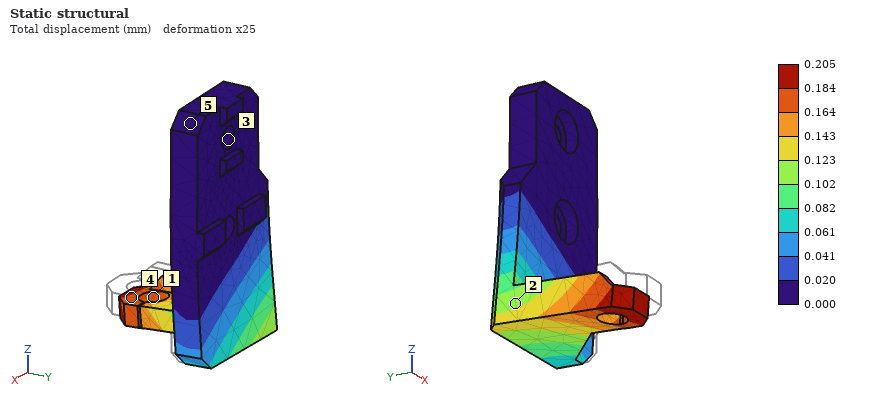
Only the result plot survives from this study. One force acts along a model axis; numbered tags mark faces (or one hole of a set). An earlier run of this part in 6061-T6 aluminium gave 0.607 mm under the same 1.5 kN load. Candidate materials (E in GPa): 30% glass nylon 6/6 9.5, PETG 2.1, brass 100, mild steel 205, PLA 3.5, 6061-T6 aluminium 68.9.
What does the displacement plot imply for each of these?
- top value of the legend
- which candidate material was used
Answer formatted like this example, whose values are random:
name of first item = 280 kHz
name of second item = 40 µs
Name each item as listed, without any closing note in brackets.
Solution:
top value of the legend = 0.205 mm
which candidate material was used = mild steel
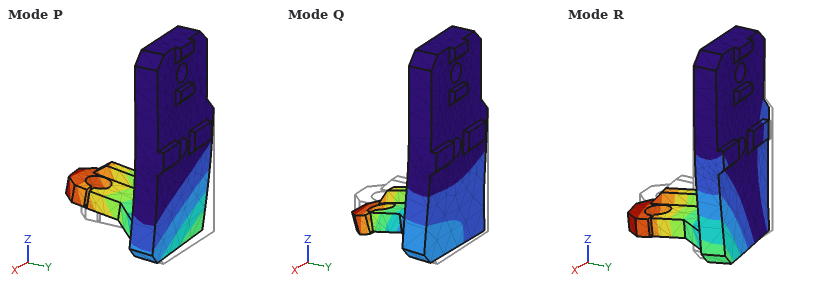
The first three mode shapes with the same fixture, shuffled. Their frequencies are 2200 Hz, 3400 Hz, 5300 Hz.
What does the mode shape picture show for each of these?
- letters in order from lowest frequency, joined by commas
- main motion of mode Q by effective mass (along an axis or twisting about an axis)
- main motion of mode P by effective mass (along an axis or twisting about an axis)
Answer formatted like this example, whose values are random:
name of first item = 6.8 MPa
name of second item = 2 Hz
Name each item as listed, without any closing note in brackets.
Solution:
letters in order from lowest frequency, joined by commas = P, R, Q
main motion of mode Q by effective mass = along Y
main motion of mode P by effective mass = along Y
